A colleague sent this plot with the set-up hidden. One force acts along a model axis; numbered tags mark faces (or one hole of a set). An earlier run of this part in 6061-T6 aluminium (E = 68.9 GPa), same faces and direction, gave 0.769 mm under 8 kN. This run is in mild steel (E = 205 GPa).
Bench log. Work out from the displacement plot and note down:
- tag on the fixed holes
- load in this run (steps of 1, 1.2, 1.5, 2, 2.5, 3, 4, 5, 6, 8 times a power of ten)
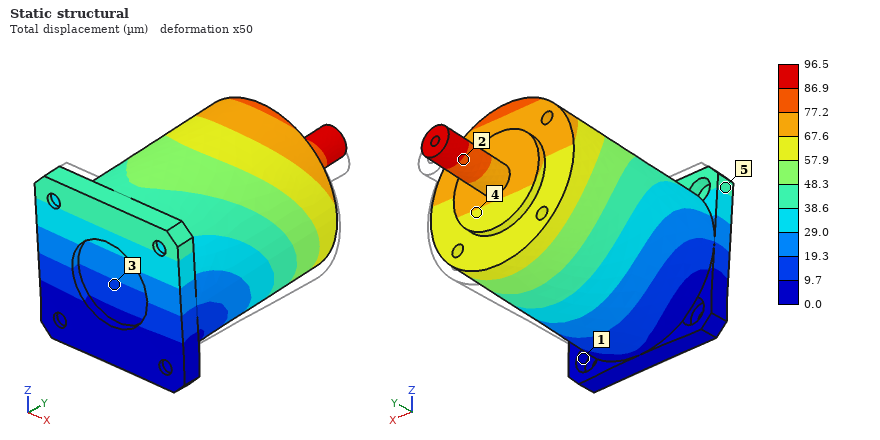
1
3 kN
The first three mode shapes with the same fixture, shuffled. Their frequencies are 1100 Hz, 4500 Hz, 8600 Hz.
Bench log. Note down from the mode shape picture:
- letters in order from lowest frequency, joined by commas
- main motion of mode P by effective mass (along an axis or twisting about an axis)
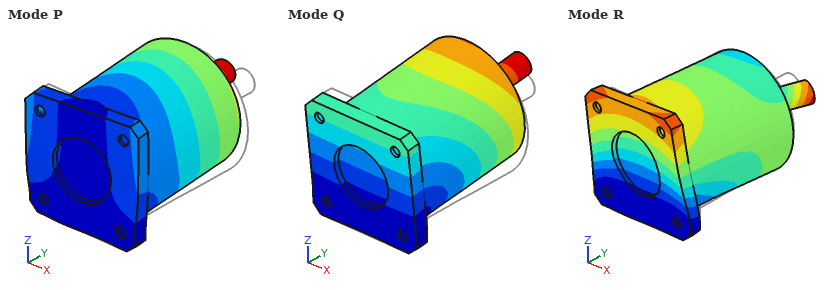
Q, P, R
along X
